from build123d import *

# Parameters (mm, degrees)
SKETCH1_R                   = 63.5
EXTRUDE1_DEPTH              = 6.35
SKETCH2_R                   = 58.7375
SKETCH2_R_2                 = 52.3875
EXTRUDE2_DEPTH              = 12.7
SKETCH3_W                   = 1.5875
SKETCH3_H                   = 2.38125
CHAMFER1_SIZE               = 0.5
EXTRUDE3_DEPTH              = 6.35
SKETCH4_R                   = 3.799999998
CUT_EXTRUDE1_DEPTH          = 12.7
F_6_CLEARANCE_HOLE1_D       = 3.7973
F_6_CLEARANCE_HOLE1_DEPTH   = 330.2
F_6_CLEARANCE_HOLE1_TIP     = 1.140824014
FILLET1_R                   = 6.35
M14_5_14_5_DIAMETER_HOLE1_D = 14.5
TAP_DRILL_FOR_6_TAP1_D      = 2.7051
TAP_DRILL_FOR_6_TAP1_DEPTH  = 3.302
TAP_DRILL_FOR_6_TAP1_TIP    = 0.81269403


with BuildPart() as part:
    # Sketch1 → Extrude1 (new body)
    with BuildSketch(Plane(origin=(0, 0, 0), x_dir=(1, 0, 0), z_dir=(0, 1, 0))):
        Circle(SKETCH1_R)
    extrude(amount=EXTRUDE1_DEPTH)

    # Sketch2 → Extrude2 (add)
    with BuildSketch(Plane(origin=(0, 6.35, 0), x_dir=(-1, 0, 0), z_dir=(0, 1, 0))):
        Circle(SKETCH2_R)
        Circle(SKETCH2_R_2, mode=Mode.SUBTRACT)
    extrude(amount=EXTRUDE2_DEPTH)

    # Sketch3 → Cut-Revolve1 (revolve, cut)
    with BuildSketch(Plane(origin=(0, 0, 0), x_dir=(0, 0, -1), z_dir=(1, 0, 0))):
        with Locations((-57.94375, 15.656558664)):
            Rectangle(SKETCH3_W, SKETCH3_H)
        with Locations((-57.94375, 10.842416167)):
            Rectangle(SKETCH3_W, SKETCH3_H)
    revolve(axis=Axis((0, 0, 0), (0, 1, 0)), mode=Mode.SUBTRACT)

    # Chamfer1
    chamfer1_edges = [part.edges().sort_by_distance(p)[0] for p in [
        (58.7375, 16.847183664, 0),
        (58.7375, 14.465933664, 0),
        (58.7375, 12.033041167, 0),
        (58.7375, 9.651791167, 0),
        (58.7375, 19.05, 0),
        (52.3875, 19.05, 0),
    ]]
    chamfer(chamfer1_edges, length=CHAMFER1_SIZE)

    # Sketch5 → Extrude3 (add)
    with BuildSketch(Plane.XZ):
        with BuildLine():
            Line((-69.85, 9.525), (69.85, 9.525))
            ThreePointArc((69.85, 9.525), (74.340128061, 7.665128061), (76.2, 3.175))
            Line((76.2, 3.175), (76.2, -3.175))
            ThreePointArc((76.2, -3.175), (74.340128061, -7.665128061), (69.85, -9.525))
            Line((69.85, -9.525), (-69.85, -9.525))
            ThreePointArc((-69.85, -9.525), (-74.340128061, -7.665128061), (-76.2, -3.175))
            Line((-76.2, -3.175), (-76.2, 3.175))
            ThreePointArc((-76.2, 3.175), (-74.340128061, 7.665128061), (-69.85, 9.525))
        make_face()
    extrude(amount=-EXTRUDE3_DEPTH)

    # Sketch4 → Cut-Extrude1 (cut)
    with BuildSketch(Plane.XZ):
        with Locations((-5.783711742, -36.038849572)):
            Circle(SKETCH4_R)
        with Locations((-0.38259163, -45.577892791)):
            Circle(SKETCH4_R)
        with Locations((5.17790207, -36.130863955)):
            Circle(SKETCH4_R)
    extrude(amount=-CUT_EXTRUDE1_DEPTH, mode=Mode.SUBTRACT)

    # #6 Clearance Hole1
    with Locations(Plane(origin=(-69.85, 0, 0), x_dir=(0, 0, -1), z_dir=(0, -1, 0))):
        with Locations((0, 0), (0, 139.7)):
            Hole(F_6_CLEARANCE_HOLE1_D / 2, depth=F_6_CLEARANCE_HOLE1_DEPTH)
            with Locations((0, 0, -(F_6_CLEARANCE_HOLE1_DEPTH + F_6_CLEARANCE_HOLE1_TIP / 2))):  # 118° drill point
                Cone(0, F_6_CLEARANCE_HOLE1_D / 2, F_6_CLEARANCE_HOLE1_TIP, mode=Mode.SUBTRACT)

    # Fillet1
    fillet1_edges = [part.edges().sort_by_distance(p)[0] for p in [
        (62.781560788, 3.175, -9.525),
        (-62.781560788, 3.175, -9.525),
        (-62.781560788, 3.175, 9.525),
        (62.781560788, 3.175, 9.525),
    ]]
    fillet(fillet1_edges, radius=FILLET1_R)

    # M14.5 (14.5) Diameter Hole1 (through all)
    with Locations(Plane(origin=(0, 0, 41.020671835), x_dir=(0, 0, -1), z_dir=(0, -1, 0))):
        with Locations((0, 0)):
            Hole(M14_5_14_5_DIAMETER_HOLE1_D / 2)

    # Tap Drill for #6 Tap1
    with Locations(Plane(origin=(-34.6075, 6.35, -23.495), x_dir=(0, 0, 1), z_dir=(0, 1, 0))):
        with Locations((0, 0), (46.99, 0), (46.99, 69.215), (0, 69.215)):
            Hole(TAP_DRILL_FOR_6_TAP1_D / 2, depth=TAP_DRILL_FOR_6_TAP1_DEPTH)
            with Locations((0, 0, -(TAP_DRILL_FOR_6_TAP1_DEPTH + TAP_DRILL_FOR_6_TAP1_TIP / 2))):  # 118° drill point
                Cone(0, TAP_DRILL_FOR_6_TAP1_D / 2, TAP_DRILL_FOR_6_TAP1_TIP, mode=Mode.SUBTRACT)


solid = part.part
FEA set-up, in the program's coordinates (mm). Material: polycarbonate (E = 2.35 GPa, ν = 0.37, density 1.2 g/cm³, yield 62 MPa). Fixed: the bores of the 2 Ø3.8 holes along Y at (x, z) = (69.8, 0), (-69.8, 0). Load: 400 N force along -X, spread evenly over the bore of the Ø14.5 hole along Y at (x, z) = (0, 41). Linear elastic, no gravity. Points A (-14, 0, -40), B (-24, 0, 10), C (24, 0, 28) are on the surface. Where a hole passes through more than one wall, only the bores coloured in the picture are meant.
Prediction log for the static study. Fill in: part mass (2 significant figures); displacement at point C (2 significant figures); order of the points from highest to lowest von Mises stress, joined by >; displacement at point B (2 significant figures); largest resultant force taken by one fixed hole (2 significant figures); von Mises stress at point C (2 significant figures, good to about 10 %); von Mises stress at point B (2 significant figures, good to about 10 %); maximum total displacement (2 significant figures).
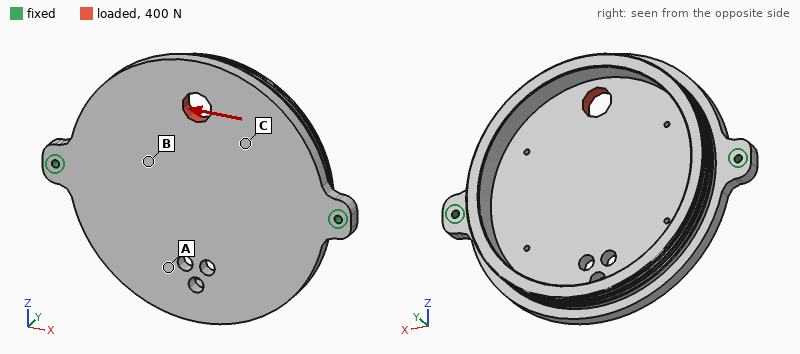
130 g
40 µm
C > B > A
26 µm
230 N
1.1 MPa
0.76 MPa
63 µm
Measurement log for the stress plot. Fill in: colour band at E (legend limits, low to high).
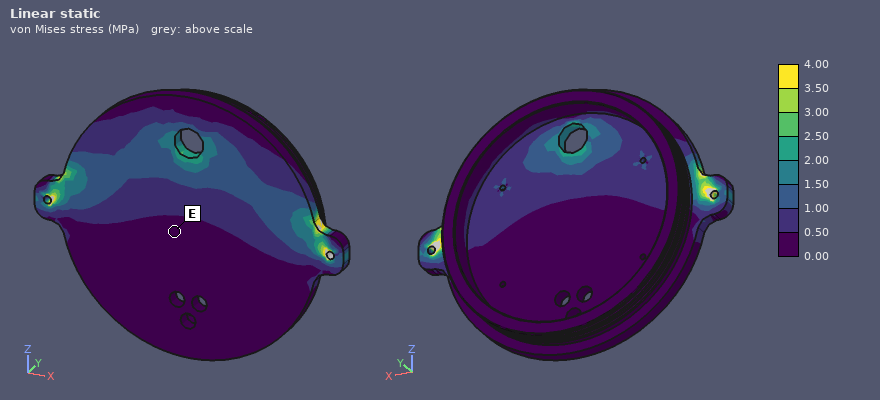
0.00 to 0.50 MPa
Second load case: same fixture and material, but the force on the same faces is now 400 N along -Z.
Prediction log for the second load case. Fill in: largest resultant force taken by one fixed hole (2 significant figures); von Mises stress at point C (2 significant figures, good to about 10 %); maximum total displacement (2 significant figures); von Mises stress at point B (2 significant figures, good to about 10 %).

200 N
0.85 MPa
77 µm
0.56 MPa
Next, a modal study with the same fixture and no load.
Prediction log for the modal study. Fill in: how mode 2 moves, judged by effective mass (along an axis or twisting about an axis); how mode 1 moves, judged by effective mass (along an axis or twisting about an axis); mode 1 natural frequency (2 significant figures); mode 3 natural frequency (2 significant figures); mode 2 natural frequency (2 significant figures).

along Y
twisting about X
180 Hz
860 Hz
330 Hz
